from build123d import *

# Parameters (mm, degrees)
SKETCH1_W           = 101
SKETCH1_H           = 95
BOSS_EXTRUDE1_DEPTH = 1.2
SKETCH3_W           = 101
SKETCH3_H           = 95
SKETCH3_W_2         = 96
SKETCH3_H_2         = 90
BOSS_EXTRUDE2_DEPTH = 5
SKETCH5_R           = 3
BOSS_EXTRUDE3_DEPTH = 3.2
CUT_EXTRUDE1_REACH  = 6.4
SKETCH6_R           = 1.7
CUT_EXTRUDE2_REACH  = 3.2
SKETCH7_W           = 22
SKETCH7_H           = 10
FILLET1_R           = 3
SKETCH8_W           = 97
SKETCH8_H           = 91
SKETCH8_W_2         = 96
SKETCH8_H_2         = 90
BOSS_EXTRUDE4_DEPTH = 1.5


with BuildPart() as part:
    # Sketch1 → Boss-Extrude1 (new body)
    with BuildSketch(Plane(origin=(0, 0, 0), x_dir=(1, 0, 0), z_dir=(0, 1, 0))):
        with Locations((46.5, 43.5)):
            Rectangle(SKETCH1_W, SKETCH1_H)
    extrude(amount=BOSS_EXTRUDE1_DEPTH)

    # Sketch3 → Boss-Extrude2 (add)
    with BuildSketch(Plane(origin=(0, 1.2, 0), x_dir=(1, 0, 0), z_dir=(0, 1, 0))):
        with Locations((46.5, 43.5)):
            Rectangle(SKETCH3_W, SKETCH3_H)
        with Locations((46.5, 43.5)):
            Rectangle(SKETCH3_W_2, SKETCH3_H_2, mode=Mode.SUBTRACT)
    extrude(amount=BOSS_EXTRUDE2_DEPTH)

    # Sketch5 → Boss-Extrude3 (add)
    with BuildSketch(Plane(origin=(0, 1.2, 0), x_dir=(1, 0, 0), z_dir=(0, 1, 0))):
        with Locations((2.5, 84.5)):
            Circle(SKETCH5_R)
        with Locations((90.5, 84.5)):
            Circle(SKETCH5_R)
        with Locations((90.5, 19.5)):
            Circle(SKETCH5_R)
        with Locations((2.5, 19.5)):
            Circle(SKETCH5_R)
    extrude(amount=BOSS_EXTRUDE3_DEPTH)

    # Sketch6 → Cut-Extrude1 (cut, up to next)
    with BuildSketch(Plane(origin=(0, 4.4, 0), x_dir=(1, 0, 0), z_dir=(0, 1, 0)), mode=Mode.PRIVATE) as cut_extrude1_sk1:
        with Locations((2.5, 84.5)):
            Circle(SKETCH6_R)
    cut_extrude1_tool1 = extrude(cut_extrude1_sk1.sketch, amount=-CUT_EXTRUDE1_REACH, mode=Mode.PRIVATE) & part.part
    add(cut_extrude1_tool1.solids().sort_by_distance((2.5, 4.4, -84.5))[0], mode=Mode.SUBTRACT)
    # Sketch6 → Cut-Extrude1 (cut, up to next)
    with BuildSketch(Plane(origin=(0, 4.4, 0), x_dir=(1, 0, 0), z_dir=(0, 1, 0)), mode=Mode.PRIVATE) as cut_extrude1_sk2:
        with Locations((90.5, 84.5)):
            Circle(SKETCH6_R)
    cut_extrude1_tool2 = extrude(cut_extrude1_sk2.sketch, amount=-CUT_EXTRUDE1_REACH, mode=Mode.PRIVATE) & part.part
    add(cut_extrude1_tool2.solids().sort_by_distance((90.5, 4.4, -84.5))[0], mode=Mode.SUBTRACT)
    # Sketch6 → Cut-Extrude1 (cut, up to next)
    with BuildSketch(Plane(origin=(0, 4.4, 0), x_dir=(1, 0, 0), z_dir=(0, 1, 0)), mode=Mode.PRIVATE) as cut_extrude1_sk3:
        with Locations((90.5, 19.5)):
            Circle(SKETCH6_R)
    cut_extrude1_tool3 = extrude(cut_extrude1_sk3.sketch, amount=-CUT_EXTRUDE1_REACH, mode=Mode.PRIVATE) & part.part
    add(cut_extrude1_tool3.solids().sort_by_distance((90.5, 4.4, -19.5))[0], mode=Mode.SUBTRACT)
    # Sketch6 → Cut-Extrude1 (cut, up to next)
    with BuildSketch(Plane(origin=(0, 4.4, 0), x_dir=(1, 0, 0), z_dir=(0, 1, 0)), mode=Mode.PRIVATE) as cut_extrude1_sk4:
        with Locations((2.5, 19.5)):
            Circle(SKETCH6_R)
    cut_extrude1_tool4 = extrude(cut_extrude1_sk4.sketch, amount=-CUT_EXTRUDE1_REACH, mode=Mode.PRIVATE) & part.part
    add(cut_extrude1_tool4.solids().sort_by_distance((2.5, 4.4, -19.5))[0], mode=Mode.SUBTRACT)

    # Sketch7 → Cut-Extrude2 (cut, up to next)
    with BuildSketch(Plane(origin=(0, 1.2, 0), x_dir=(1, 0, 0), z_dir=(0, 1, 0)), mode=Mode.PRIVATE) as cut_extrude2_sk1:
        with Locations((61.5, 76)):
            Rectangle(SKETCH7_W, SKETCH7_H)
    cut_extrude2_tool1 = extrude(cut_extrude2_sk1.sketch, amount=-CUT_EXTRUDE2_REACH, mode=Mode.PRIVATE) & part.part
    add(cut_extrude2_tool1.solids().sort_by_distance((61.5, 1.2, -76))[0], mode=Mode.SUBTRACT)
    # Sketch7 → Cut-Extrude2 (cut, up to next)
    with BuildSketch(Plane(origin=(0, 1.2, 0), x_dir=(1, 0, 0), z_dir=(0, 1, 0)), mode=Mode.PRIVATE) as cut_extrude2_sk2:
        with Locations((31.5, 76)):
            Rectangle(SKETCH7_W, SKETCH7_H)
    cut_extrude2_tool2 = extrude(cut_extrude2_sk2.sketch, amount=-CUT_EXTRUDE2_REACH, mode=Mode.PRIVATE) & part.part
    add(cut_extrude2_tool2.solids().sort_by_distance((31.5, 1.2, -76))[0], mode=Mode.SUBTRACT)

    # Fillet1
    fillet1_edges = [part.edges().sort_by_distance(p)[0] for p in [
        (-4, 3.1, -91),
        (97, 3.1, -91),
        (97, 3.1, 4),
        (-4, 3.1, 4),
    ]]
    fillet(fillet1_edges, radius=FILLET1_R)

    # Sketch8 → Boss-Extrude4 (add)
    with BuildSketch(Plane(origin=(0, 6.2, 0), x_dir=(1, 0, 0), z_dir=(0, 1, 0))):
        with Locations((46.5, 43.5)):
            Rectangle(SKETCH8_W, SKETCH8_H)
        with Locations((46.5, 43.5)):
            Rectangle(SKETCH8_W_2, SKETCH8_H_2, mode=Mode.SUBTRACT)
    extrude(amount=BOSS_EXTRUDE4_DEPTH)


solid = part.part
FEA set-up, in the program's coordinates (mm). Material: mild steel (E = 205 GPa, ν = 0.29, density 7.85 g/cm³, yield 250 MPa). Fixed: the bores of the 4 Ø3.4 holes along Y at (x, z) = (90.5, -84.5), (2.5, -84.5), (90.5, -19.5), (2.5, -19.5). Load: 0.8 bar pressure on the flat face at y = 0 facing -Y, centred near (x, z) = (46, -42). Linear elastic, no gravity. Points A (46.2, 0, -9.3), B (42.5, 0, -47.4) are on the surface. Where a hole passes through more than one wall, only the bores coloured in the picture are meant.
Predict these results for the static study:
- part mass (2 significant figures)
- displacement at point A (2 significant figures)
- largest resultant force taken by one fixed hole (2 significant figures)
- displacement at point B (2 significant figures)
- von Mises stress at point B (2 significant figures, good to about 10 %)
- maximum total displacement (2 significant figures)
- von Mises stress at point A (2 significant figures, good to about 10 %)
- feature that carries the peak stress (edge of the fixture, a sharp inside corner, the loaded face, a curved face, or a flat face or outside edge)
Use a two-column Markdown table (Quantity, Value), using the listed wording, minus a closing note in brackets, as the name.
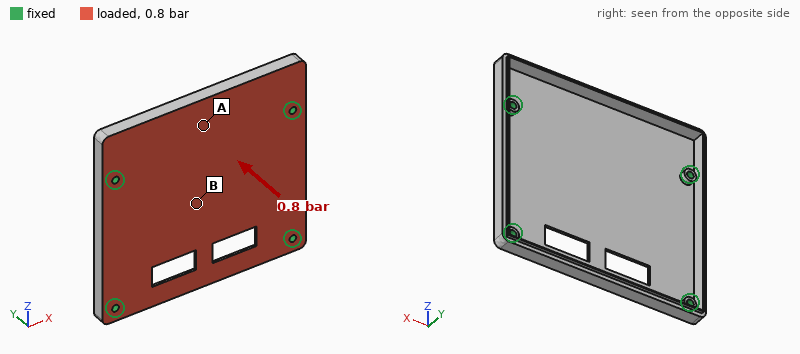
| Quantity | Value |
|---|---|
| part mass | 130 g |
| displacement at point A | 0.17 mm |
| largest resultant force taken by one fixed hole | 240 N |
| displacement at point B | 0.36 mm |
| von Mises stress at point B | 79 MPa |
| maximum total displacement | 0.36 mm |
| von Mises stress at point A | 40 MPa |
| feature that carries the peak stress | the loaded face |
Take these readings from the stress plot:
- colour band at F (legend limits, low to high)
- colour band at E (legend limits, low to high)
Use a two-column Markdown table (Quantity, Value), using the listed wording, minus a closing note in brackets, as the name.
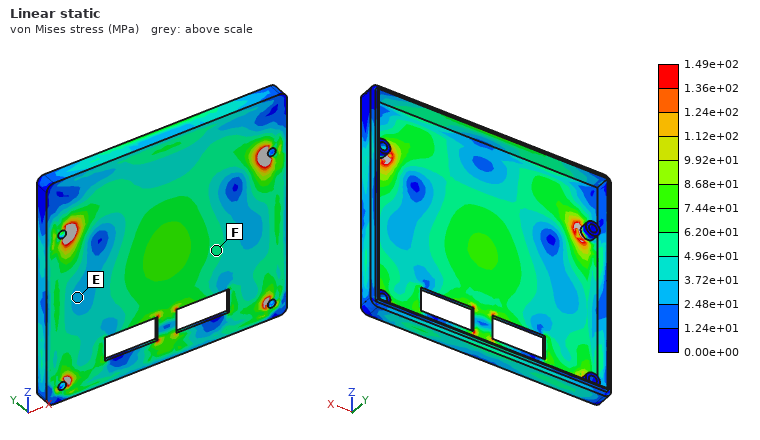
| Quantity | Value |
|---|---|
| colour band at F | 4.96e+01 to 6.20e+01 MPa |
| colour band at E | 2.48e+01 to 3.72e+01 MPa |
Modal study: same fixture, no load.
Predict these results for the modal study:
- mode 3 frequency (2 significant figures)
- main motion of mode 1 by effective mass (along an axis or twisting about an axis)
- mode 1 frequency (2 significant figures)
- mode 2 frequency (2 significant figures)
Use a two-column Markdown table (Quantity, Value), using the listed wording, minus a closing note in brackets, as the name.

| Quantity | Value |
|---|---|
| mode 3 frequency | 2000 Hz |
| main motion of mode 1 by effective mass | along Y |
| mode 1 frequency | 960 Hz |
| mode 2 frequency | 1500 Hz |
